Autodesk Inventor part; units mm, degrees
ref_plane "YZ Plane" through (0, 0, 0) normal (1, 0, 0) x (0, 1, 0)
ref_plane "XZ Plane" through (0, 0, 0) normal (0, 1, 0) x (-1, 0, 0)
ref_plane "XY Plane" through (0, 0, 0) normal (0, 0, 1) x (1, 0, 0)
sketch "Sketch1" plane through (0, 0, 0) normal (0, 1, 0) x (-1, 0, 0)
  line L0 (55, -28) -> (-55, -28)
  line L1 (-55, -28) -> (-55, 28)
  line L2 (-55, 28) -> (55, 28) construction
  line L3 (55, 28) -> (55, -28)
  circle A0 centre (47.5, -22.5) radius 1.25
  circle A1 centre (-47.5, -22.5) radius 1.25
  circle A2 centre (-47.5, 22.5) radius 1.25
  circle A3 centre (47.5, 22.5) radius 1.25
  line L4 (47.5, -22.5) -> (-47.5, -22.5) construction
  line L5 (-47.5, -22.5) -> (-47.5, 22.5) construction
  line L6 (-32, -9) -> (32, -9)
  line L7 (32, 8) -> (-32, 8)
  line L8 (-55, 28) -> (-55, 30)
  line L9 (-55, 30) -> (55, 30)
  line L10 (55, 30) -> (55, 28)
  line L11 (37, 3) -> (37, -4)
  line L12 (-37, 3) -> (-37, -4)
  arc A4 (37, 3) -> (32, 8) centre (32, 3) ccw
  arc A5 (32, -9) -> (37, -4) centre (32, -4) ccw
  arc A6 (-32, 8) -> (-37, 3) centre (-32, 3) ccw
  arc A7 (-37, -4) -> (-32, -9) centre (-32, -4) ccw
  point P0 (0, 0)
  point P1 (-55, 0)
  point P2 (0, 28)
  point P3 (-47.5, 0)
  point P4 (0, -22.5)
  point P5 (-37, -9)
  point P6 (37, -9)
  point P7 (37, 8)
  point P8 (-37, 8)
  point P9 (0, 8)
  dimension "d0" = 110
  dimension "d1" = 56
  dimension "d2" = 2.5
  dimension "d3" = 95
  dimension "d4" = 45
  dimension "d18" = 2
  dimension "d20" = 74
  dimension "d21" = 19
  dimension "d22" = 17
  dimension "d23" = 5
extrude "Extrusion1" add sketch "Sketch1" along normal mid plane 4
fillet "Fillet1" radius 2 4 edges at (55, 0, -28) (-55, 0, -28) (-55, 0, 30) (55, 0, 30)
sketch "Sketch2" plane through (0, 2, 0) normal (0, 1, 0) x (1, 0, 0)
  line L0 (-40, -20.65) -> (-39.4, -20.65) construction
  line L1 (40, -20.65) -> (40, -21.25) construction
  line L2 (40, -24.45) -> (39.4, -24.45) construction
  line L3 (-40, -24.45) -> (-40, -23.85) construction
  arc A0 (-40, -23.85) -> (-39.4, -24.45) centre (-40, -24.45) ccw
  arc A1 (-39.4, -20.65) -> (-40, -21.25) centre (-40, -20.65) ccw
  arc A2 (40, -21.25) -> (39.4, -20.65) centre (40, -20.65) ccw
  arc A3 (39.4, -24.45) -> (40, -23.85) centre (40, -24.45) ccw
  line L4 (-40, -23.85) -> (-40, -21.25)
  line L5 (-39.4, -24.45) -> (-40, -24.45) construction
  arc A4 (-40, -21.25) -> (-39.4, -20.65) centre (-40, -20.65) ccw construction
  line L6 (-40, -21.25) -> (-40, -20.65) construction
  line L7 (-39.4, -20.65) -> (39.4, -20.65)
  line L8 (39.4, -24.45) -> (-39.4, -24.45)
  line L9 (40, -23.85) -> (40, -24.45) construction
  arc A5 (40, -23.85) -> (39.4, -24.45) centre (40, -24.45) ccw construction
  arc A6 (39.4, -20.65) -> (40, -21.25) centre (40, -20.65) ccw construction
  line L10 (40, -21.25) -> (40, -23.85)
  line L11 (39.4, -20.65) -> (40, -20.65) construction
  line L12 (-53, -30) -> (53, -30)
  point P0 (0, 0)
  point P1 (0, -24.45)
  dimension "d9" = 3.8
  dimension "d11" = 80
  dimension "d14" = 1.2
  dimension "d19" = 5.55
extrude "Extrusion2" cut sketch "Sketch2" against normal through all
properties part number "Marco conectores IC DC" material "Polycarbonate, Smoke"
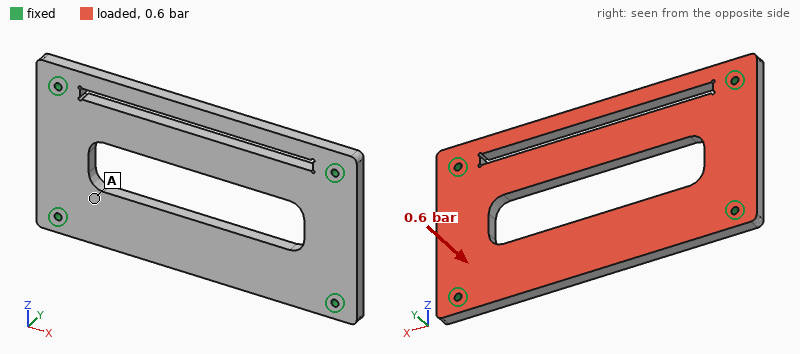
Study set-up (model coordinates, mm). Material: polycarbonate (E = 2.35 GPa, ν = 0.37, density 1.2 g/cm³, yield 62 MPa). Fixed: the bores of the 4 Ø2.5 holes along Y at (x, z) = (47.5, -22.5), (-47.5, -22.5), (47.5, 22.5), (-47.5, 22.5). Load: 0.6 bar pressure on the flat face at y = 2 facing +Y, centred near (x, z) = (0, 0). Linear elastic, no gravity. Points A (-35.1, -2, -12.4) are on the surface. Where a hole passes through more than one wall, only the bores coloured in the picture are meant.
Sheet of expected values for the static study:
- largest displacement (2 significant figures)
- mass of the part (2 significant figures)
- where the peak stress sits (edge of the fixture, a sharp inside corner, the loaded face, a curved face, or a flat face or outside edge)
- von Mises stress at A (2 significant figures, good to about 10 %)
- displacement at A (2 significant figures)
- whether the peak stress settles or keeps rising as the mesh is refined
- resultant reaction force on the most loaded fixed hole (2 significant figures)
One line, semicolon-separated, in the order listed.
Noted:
1.3 mm; 23 g; edge of the fixture; 4.6 MPa; 0.38 mm; keeps rising; 73 N
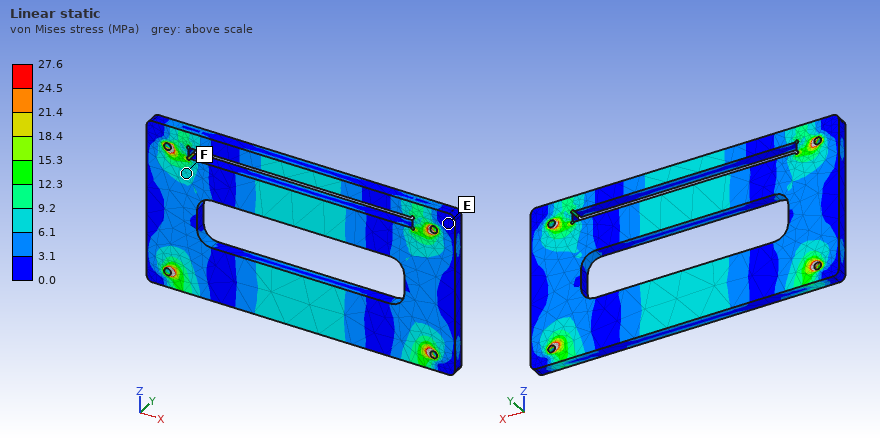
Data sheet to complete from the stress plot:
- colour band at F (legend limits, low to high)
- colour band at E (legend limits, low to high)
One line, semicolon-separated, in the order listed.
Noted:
6.1 to 9.2 MPa; 0.0 to 3.1 MPa
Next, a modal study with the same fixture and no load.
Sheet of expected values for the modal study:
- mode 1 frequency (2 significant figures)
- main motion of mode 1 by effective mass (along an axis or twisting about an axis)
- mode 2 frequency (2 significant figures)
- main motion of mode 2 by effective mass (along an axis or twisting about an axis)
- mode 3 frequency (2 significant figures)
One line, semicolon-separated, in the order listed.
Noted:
590 Hz; along Y; 650 Hz; twisting about X; 680 Hz
